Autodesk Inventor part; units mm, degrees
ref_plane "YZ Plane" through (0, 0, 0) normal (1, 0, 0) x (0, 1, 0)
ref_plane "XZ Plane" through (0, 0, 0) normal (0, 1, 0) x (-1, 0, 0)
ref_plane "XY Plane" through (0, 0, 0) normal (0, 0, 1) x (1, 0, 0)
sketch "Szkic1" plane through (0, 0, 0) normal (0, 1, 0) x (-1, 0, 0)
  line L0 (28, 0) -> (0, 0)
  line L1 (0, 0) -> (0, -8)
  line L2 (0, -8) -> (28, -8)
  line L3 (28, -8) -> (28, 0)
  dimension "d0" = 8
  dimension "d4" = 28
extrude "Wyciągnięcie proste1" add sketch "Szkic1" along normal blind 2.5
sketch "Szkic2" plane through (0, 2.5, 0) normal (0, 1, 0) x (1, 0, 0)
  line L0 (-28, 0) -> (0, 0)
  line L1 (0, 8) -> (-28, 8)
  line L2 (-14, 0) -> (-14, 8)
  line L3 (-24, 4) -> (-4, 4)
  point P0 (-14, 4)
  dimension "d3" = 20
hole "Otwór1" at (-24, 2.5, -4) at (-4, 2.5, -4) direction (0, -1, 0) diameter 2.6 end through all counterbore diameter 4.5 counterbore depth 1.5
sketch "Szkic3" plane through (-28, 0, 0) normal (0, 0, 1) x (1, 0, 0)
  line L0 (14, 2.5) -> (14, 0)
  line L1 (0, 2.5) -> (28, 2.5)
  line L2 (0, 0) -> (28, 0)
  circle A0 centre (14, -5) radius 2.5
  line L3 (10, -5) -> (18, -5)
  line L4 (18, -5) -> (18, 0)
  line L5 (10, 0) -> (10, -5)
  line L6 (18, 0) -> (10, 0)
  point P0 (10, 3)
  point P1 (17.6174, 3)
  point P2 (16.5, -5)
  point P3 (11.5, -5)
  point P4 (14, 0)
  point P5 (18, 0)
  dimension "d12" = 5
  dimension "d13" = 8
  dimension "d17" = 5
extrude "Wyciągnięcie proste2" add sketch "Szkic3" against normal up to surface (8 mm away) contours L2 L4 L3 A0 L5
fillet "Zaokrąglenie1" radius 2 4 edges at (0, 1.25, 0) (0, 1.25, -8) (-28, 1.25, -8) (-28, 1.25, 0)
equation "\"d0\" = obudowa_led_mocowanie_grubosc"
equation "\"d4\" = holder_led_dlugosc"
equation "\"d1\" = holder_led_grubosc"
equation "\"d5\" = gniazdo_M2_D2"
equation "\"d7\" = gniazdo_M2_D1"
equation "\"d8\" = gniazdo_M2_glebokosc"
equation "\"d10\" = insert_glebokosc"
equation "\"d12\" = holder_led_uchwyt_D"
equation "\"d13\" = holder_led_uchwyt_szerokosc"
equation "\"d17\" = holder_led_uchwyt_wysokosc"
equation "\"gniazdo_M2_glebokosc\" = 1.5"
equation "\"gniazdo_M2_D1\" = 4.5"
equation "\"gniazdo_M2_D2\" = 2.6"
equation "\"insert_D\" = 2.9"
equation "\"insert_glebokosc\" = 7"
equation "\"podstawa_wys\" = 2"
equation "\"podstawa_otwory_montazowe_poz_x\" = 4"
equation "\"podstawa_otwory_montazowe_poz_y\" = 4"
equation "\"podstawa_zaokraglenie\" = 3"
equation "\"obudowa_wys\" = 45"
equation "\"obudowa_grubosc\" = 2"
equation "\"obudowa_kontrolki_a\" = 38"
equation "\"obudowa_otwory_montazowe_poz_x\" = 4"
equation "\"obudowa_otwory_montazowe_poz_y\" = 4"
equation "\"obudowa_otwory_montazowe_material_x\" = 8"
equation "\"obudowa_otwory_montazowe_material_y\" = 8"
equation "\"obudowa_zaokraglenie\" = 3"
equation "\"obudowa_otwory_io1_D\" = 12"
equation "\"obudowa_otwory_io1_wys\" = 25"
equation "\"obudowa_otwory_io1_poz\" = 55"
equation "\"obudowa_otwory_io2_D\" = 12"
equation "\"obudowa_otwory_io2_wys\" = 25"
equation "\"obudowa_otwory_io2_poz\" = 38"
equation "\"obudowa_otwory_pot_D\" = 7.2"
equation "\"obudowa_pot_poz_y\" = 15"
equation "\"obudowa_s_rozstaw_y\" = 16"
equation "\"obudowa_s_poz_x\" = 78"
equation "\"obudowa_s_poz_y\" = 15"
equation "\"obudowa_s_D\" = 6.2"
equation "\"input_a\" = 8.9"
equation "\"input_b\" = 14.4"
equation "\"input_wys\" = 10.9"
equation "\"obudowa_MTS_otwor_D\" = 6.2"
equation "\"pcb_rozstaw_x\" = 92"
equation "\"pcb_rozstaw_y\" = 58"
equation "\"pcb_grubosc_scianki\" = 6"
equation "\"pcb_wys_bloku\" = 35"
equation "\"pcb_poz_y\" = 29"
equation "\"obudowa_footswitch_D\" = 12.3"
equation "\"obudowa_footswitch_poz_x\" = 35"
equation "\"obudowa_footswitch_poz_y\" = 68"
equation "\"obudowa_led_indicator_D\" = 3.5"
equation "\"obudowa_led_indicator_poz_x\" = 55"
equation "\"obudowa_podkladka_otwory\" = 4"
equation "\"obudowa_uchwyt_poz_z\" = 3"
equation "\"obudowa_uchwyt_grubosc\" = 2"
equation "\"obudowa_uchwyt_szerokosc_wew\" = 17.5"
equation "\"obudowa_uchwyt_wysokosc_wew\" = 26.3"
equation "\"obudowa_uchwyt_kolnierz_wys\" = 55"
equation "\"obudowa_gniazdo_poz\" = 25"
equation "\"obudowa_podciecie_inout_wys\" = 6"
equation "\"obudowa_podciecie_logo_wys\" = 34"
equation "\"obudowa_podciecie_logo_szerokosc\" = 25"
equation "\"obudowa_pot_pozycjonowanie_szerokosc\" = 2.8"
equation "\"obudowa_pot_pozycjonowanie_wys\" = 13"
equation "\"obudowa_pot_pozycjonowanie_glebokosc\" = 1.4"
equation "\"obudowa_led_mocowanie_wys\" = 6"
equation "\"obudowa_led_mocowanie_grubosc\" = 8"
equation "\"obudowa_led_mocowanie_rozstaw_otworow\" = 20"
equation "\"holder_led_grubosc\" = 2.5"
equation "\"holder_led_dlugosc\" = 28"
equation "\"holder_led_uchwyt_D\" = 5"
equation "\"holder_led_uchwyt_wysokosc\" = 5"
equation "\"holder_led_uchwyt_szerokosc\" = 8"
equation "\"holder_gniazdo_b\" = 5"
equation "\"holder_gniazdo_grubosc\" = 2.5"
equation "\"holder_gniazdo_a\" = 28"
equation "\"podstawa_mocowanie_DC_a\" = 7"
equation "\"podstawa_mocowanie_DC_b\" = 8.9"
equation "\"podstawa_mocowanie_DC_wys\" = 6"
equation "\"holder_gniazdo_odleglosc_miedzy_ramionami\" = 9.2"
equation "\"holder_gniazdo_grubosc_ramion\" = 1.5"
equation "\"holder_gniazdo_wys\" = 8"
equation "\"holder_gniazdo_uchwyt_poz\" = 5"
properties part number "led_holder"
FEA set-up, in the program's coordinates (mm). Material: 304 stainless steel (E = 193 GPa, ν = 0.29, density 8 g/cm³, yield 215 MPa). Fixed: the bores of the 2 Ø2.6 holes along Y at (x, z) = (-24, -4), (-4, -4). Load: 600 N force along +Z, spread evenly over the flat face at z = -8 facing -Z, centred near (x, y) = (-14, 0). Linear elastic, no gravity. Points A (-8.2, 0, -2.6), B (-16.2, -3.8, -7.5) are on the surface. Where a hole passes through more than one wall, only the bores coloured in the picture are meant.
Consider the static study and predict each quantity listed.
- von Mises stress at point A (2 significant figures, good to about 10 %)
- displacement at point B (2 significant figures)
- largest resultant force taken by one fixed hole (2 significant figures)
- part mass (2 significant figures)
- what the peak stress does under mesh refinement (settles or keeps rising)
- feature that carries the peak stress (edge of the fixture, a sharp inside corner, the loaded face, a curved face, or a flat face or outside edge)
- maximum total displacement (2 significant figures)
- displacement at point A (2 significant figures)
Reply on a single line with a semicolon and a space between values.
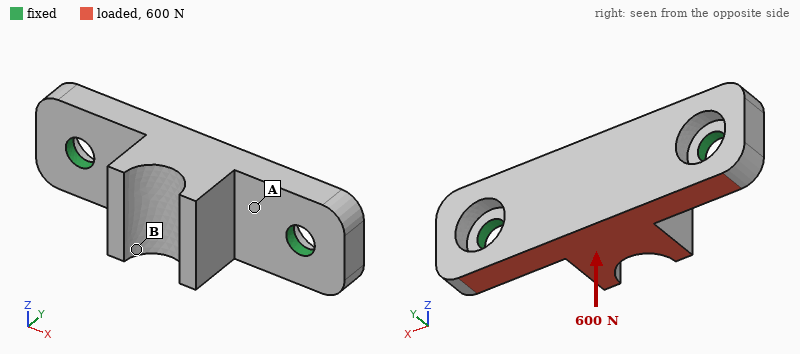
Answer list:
53 MPa; 7.0 µm; 300 N; 5.9 g; keeps rising; edge of the fixture; 7.9 µm; 2.3 µm
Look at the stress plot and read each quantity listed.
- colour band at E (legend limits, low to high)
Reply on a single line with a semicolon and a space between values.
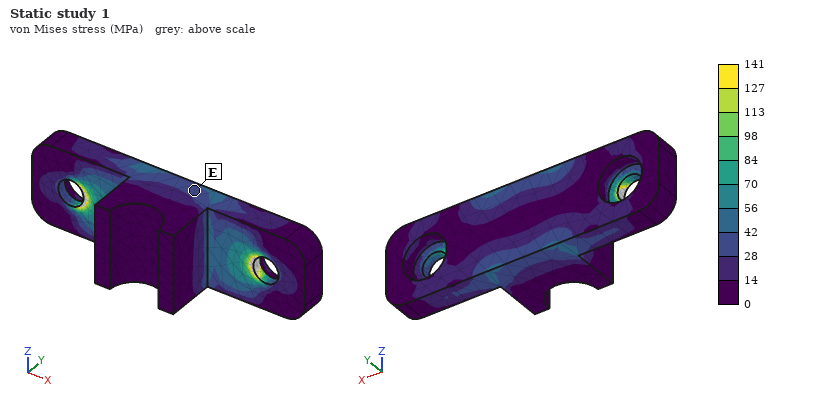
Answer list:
28 to 42 MPa
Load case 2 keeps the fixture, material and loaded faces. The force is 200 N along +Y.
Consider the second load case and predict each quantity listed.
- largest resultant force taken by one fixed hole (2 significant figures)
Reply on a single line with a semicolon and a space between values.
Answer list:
110 N
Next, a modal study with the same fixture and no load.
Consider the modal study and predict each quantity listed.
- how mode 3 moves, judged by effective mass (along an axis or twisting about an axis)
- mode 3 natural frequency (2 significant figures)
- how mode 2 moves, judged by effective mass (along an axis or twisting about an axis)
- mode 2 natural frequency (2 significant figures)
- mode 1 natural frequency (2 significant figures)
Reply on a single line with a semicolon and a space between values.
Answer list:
along Z; 33 kHz; along Y; 20 kHz; 17 kHz
